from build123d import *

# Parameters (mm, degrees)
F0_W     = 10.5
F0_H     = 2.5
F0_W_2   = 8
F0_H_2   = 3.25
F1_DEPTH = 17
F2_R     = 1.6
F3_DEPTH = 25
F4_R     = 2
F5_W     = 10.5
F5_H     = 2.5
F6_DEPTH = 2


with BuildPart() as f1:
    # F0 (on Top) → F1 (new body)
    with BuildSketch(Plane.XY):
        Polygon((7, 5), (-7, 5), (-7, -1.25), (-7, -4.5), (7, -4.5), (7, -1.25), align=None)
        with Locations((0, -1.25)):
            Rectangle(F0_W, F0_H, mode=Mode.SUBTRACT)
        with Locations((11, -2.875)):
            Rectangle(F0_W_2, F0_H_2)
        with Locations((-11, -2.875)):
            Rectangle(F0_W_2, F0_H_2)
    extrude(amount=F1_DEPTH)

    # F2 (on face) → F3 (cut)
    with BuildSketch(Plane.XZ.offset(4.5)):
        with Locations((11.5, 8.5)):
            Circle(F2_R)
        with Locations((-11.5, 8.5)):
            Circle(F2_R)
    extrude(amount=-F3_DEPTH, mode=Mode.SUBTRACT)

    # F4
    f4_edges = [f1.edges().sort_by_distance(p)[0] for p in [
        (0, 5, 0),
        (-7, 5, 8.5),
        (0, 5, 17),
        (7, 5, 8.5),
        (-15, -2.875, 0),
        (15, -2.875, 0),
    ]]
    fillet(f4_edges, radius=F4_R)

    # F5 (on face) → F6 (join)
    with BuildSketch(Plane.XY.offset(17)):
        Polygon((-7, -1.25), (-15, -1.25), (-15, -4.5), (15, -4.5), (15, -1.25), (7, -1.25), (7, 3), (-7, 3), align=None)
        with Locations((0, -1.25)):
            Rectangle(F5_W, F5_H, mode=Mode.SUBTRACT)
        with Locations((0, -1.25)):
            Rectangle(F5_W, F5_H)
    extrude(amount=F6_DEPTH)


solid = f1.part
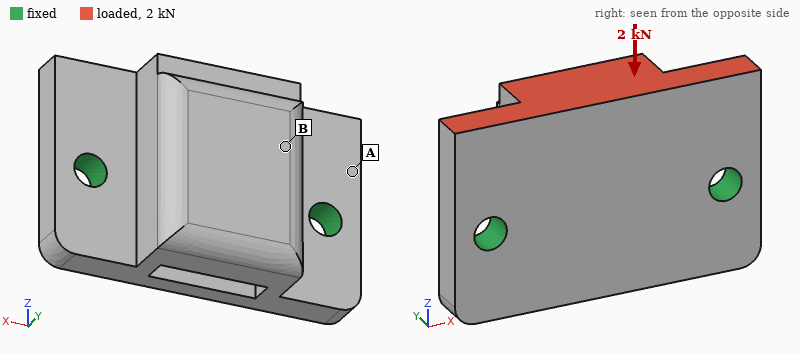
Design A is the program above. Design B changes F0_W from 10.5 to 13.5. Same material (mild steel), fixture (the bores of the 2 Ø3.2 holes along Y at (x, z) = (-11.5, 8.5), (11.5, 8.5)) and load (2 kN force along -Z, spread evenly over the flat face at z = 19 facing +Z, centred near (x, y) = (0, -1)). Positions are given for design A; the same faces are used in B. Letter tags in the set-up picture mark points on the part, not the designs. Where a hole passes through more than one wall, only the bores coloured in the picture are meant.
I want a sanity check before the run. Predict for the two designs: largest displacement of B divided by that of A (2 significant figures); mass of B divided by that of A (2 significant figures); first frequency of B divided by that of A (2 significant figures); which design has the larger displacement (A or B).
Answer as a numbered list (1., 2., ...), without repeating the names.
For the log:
1. 1.3
2. 0.96
3. 0.93
4. B
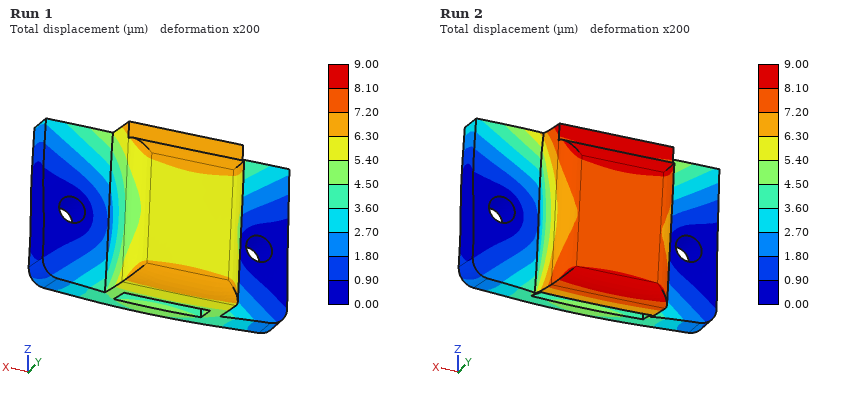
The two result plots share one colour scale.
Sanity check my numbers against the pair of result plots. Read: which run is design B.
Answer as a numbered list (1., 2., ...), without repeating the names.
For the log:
1. Run 2
